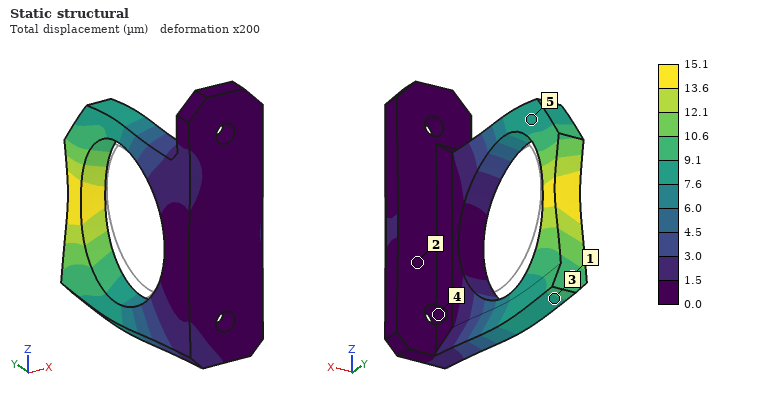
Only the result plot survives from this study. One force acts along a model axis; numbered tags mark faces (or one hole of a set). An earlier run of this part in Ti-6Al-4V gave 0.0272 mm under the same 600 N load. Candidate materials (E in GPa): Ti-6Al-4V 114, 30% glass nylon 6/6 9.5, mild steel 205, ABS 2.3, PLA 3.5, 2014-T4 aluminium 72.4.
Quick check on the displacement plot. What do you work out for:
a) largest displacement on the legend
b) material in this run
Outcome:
15.1 µm
mild steel
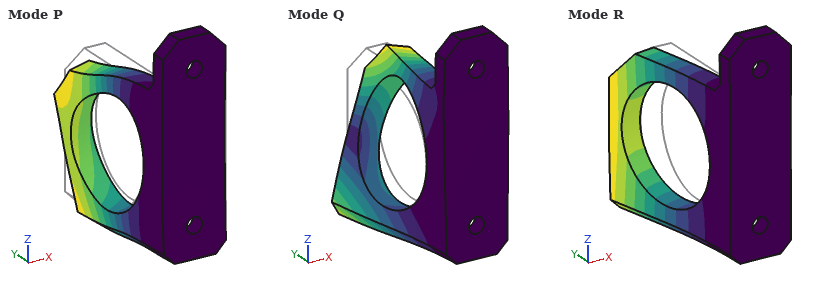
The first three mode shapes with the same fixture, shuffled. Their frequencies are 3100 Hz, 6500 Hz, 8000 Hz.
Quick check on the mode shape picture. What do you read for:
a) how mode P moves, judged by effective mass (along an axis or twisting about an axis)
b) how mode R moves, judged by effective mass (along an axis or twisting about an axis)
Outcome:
along Z
along X
